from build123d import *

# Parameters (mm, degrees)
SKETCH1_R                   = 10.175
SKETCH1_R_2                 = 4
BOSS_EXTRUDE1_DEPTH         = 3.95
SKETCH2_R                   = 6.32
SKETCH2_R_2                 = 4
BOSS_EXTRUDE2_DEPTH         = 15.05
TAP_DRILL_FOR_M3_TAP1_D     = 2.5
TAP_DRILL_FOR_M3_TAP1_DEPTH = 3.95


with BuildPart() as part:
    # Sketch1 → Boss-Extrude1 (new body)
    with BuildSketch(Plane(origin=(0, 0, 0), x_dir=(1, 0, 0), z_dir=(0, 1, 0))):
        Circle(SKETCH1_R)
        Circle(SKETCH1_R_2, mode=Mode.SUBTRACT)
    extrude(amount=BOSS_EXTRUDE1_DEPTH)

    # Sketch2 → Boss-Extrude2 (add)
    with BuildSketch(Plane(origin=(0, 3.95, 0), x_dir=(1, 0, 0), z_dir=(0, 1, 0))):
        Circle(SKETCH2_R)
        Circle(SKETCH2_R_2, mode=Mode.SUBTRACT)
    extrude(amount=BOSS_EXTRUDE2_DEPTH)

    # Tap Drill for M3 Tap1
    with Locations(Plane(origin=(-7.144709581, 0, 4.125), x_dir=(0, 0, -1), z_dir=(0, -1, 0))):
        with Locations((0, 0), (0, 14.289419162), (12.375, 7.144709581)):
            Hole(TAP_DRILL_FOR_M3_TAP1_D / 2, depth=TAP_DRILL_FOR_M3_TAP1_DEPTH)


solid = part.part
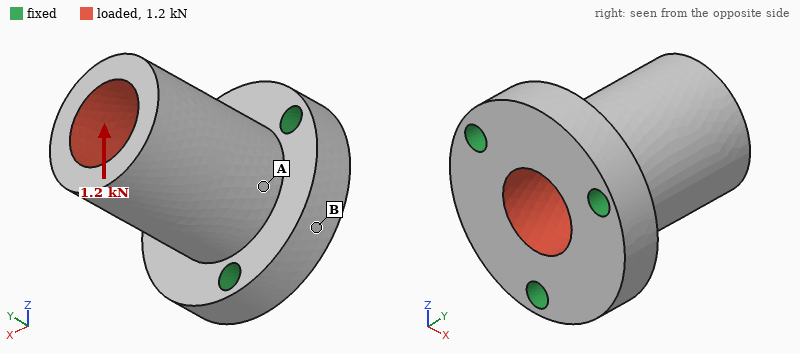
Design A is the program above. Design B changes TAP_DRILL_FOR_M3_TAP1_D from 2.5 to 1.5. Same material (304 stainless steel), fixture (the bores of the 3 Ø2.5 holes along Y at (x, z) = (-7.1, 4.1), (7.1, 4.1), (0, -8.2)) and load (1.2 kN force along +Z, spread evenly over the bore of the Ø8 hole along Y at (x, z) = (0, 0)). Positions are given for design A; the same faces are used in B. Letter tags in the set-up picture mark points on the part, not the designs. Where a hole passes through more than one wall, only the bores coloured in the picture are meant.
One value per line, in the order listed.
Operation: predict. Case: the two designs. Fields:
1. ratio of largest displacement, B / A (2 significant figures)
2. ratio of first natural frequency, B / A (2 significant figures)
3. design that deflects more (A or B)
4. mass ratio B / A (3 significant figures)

1.2
0.93
B
1.02
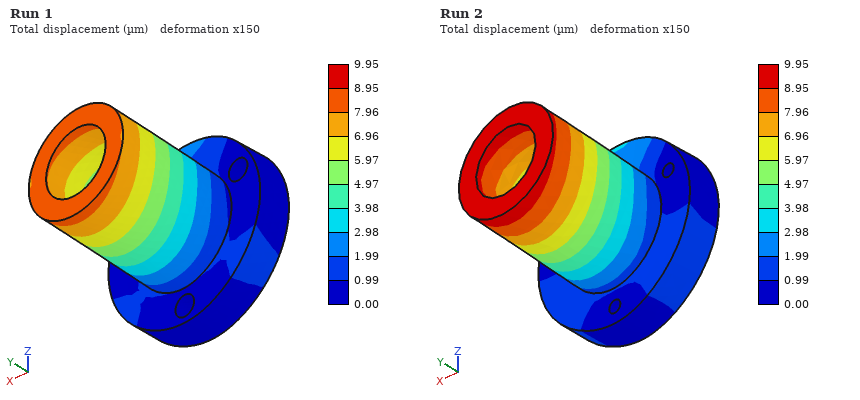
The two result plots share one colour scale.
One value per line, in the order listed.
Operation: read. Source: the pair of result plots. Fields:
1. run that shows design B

Run 2
